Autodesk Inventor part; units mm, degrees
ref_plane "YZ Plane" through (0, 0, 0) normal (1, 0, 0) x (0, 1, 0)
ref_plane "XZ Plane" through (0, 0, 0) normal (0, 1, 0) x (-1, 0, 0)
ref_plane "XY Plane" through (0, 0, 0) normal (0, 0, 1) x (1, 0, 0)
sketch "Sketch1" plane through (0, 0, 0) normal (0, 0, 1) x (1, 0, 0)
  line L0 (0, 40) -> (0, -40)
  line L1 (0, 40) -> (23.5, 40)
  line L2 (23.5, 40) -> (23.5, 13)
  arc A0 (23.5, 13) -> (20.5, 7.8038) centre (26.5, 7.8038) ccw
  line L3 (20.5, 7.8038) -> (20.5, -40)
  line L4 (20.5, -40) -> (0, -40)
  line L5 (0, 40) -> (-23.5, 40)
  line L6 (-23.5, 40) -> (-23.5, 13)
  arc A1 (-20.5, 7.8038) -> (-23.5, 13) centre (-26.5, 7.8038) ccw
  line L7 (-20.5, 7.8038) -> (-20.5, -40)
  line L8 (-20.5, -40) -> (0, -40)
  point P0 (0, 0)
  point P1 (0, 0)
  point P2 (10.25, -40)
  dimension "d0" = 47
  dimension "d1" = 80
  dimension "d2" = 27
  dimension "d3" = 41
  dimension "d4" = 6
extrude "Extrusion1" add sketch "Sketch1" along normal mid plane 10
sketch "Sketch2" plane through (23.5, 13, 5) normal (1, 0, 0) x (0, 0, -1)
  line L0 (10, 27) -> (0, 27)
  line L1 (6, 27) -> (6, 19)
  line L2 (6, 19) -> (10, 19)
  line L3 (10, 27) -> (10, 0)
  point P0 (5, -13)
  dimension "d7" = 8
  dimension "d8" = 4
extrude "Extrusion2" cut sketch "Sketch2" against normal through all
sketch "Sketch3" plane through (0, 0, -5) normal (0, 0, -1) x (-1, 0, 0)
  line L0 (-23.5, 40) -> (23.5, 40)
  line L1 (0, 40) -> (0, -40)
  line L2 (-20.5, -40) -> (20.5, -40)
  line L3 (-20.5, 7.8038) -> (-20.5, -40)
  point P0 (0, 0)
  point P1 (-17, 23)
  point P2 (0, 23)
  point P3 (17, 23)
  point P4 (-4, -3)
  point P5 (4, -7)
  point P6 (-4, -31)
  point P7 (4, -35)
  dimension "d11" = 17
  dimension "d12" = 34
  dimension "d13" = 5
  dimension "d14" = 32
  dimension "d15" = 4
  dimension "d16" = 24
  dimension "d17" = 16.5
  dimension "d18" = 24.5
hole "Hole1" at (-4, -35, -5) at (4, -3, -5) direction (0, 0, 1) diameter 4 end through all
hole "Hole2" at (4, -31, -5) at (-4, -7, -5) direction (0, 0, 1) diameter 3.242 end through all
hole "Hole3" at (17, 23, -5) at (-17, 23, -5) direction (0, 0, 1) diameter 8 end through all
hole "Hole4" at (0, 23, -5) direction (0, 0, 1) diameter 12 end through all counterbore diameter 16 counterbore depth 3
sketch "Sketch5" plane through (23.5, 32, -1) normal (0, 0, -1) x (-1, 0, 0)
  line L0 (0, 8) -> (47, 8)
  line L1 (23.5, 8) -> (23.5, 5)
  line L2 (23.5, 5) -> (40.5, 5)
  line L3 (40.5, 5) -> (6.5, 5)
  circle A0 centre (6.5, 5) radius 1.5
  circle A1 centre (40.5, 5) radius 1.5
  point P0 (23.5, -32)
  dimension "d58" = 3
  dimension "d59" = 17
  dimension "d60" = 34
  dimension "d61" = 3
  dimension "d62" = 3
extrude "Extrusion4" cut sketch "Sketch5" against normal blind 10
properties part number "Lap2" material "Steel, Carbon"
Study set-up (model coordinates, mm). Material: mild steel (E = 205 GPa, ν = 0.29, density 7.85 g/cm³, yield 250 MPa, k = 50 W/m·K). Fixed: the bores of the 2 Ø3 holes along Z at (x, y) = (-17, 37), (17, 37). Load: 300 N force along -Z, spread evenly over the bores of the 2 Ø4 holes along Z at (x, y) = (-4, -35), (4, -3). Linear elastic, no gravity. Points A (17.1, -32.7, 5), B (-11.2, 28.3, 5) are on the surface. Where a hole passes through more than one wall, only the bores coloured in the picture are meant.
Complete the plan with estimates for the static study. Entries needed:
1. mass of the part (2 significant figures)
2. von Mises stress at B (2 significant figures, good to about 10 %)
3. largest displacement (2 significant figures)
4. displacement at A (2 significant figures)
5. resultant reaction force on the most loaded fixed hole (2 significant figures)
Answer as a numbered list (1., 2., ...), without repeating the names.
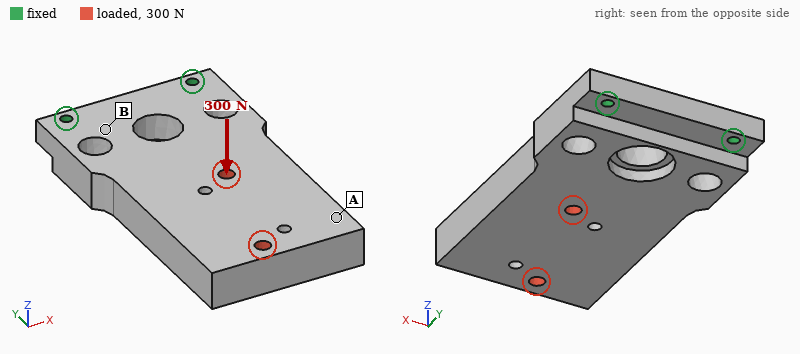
1. 240 g
2. 42 MPa
3. 0.13 mm
4. 0.12 mm
5. 160 N
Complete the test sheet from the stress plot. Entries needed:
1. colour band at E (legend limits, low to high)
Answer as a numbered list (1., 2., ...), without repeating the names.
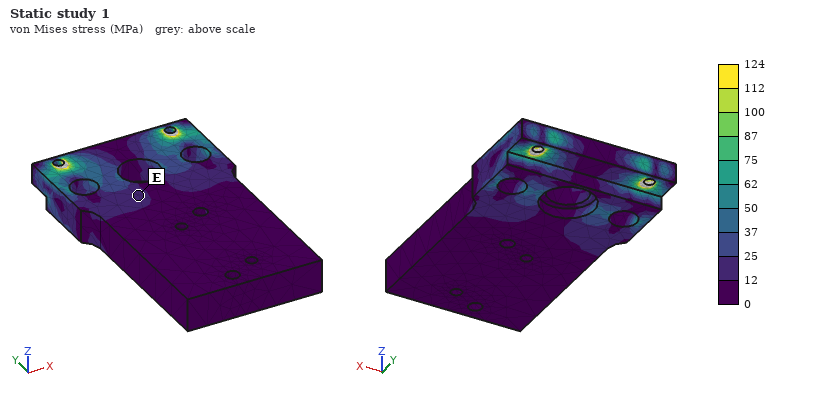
1. 12 to 25 MPa
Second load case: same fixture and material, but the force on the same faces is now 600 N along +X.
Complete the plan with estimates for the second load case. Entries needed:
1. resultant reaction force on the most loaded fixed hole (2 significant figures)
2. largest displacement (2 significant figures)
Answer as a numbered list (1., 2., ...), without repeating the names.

1. 990 N
2. 9.9 µm
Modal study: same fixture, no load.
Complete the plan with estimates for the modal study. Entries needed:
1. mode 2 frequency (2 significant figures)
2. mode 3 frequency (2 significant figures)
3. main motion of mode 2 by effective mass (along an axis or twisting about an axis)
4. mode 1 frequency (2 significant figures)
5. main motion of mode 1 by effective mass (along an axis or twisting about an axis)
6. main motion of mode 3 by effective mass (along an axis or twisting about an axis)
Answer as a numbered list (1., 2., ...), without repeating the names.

1. 3700 Hz
2. 4300 Hz
3. along X
4. 750 Hz
5. along Z
6. along X
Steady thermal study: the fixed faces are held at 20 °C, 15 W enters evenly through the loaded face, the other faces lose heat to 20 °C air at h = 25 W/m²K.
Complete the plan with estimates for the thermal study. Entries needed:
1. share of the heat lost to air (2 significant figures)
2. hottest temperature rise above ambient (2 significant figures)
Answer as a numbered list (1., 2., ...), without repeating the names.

1. 39 %
2. 43 K
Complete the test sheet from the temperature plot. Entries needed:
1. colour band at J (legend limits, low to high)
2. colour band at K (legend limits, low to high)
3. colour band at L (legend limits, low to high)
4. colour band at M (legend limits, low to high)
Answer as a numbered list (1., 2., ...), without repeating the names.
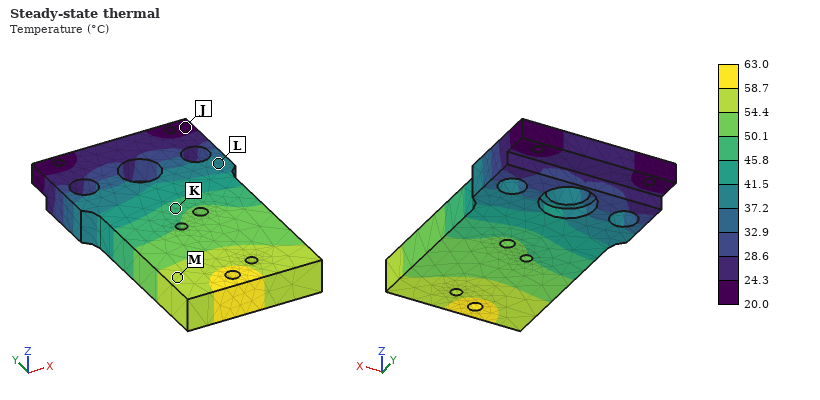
1. 20.0 to 24.3 °C
2. 45.8 to 50.1 °C
3. 37.2 to 41.5 °C
4. 54.4 to 58.7 °C
